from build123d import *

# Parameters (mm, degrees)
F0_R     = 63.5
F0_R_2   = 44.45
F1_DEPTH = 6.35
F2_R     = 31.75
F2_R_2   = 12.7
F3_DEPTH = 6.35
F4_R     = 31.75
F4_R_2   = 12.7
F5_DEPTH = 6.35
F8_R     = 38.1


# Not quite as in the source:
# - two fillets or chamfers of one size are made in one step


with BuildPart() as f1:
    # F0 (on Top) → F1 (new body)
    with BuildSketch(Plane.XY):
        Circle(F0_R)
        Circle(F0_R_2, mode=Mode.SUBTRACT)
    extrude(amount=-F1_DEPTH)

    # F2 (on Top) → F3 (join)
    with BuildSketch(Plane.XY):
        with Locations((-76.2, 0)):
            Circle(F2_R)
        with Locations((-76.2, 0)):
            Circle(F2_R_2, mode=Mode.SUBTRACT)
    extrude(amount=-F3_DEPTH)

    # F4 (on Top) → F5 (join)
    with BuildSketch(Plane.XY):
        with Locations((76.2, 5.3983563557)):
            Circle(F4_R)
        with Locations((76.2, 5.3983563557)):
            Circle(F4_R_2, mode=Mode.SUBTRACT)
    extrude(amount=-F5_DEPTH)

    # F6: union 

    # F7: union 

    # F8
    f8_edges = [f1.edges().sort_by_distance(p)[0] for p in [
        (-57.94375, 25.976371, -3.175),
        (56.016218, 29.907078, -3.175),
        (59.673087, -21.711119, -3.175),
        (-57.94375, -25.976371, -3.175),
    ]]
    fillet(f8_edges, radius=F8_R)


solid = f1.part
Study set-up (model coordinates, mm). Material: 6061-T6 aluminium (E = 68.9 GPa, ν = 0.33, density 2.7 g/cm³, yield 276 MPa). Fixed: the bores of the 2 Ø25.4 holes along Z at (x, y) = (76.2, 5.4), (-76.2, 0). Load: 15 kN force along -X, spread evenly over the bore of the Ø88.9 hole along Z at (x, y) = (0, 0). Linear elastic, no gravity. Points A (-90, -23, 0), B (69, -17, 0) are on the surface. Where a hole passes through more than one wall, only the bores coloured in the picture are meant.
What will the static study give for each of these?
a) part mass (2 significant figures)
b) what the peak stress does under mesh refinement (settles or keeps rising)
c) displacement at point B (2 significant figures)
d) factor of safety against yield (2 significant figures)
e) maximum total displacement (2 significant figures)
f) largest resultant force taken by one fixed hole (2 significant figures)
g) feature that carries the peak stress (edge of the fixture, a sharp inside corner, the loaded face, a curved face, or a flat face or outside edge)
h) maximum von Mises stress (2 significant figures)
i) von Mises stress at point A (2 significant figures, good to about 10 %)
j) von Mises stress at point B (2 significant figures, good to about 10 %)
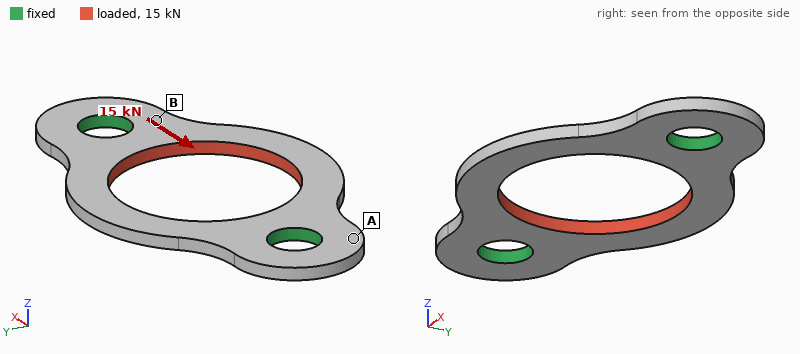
180 g
settles
7.6 µm
5.1
46 µm
7.5 kN
the loaded face
54 MPa
10 MPa
24 MPa
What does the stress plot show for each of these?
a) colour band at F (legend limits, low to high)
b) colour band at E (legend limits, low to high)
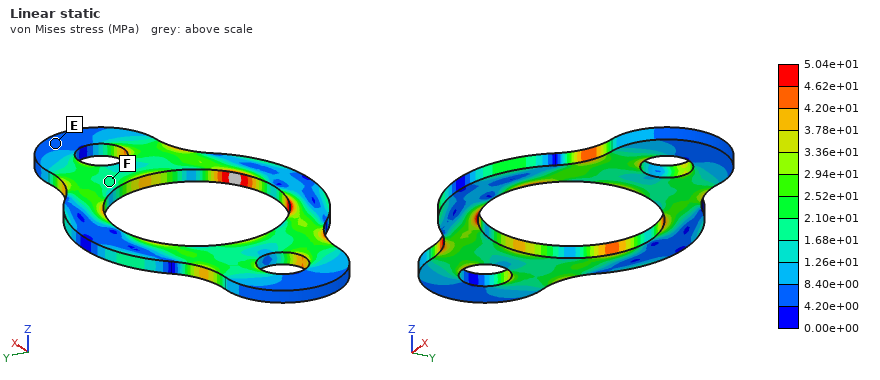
1.68e+01 to 2.10e+01 MPa
4.20e+00 to 8.40e+00 MPa
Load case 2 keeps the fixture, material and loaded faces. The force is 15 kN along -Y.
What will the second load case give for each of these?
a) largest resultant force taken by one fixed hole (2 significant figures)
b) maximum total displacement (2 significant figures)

7.5 kN
47 µm
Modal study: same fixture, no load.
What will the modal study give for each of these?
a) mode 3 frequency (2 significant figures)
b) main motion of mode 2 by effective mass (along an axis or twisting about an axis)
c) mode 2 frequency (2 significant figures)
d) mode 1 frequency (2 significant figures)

3100 Hz
along Z
1300 Hz
1100 Hz
